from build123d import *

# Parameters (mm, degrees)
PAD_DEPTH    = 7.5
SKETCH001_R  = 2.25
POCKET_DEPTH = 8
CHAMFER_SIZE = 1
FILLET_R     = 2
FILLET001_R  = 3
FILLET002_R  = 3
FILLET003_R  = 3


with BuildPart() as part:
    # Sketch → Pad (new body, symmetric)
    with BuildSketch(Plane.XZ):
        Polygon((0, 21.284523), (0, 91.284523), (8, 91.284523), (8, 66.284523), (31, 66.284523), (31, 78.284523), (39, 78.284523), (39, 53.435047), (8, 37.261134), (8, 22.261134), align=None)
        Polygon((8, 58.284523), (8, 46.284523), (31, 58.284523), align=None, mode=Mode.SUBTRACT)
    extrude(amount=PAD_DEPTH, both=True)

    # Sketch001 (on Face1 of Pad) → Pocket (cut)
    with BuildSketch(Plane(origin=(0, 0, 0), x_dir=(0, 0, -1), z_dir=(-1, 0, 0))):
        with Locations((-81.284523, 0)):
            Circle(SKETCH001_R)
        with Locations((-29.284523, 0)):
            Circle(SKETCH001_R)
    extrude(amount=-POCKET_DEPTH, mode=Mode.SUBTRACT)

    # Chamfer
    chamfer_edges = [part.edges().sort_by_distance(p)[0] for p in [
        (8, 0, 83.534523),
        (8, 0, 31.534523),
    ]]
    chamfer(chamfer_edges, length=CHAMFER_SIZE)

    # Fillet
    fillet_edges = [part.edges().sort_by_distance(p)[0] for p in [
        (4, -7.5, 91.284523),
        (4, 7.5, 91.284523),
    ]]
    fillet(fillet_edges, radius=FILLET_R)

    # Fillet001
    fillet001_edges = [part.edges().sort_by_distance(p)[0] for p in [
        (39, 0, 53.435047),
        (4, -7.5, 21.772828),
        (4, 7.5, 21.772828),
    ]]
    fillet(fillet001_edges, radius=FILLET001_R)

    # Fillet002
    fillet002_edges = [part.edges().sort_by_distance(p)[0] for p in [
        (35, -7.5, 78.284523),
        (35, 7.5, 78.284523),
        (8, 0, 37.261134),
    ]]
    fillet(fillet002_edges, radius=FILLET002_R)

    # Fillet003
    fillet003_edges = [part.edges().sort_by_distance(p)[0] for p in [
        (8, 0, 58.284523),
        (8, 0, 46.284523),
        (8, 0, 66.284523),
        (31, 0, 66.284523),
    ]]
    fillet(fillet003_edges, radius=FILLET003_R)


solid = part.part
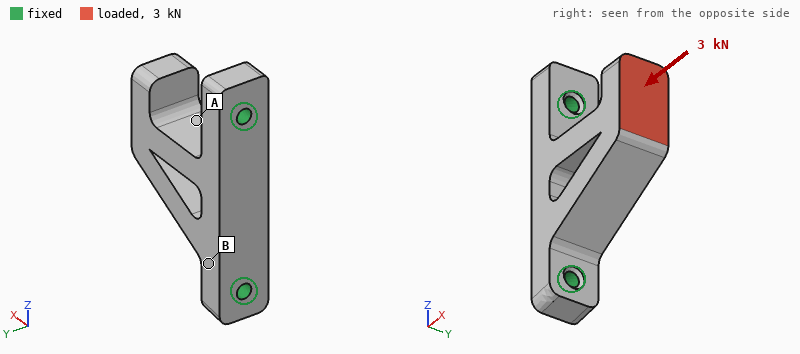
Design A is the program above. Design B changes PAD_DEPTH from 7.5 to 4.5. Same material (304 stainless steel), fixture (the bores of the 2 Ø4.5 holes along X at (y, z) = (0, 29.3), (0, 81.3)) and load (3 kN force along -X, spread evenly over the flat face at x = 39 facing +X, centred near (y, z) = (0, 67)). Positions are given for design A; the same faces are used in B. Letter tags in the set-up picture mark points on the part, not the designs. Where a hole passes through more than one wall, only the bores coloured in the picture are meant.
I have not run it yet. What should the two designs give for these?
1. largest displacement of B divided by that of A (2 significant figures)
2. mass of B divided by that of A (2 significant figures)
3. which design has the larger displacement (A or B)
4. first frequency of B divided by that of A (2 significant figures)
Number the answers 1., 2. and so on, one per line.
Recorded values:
1. 1.6
2. 0.59
3. B
4. 0.81
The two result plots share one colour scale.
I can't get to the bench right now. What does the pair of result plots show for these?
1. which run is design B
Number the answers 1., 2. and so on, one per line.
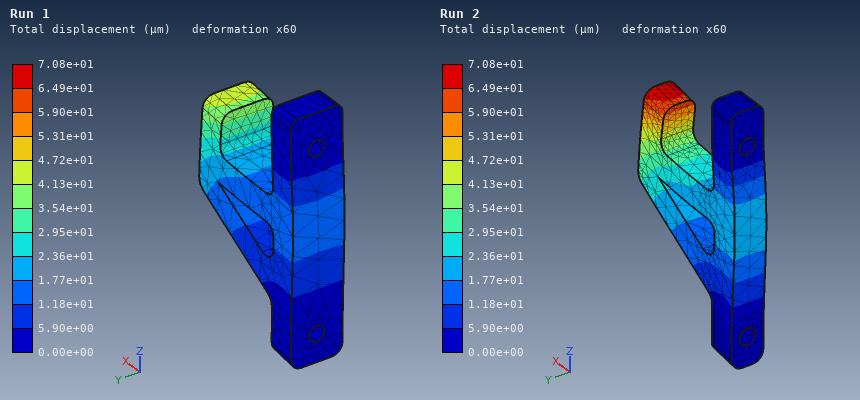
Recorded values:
1. Run 2
